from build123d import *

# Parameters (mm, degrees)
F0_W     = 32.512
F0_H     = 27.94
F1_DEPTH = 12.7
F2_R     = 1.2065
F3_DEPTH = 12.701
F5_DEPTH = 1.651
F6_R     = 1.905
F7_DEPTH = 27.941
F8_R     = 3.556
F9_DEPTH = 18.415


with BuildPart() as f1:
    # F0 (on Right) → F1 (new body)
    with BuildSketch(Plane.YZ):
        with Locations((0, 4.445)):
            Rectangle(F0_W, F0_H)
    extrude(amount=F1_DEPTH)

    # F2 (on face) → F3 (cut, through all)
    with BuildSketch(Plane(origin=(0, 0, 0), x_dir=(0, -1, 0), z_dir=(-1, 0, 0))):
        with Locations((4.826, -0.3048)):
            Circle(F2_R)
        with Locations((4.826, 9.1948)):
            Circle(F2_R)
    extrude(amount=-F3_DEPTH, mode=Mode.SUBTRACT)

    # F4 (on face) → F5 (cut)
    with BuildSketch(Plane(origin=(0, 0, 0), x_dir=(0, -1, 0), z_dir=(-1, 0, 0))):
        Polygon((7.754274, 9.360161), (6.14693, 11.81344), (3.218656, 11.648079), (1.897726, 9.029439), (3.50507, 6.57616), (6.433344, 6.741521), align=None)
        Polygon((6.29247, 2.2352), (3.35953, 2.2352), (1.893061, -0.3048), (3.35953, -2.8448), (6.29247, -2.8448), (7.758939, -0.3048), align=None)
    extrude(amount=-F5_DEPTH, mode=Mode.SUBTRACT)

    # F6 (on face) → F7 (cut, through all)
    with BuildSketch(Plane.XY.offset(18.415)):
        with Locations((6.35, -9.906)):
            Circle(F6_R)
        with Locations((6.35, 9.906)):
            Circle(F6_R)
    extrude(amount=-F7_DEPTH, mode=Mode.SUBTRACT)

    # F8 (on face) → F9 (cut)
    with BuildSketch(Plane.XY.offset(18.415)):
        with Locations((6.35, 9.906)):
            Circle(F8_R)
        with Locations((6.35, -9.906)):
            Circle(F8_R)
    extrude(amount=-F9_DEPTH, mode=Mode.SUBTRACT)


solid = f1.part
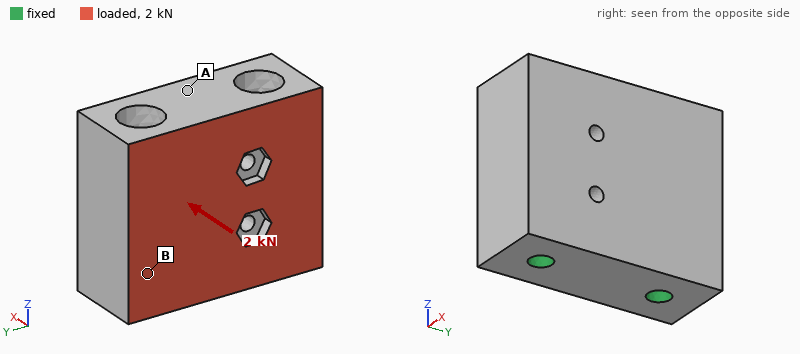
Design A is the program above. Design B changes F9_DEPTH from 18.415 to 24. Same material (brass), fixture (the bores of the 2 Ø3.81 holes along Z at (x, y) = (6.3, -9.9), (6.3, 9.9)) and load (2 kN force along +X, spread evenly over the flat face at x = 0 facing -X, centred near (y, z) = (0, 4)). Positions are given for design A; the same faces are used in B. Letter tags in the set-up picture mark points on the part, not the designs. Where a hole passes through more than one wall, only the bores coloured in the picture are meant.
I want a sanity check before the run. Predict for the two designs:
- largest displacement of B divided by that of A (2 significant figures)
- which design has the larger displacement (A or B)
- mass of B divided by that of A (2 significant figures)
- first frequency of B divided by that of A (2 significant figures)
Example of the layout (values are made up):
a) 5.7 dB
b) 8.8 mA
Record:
a) 4.7
b) B
c) 0.97
d) 0.46
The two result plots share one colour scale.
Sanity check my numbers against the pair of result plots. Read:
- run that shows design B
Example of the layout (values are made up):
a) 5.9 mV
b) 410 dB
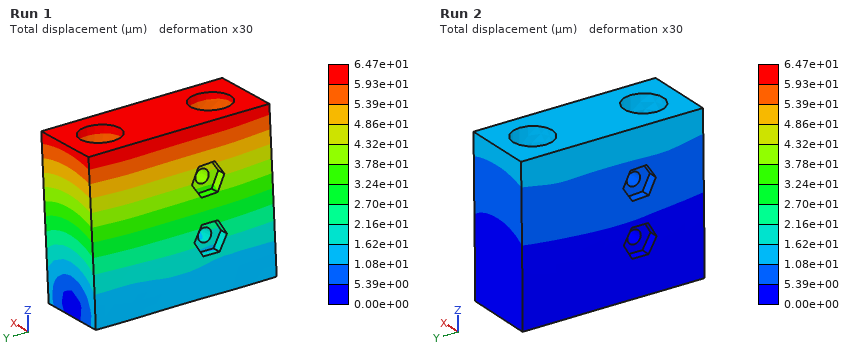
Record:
a) Run 1
